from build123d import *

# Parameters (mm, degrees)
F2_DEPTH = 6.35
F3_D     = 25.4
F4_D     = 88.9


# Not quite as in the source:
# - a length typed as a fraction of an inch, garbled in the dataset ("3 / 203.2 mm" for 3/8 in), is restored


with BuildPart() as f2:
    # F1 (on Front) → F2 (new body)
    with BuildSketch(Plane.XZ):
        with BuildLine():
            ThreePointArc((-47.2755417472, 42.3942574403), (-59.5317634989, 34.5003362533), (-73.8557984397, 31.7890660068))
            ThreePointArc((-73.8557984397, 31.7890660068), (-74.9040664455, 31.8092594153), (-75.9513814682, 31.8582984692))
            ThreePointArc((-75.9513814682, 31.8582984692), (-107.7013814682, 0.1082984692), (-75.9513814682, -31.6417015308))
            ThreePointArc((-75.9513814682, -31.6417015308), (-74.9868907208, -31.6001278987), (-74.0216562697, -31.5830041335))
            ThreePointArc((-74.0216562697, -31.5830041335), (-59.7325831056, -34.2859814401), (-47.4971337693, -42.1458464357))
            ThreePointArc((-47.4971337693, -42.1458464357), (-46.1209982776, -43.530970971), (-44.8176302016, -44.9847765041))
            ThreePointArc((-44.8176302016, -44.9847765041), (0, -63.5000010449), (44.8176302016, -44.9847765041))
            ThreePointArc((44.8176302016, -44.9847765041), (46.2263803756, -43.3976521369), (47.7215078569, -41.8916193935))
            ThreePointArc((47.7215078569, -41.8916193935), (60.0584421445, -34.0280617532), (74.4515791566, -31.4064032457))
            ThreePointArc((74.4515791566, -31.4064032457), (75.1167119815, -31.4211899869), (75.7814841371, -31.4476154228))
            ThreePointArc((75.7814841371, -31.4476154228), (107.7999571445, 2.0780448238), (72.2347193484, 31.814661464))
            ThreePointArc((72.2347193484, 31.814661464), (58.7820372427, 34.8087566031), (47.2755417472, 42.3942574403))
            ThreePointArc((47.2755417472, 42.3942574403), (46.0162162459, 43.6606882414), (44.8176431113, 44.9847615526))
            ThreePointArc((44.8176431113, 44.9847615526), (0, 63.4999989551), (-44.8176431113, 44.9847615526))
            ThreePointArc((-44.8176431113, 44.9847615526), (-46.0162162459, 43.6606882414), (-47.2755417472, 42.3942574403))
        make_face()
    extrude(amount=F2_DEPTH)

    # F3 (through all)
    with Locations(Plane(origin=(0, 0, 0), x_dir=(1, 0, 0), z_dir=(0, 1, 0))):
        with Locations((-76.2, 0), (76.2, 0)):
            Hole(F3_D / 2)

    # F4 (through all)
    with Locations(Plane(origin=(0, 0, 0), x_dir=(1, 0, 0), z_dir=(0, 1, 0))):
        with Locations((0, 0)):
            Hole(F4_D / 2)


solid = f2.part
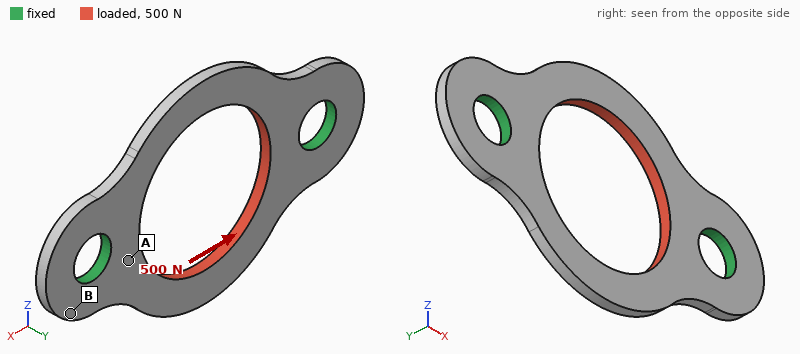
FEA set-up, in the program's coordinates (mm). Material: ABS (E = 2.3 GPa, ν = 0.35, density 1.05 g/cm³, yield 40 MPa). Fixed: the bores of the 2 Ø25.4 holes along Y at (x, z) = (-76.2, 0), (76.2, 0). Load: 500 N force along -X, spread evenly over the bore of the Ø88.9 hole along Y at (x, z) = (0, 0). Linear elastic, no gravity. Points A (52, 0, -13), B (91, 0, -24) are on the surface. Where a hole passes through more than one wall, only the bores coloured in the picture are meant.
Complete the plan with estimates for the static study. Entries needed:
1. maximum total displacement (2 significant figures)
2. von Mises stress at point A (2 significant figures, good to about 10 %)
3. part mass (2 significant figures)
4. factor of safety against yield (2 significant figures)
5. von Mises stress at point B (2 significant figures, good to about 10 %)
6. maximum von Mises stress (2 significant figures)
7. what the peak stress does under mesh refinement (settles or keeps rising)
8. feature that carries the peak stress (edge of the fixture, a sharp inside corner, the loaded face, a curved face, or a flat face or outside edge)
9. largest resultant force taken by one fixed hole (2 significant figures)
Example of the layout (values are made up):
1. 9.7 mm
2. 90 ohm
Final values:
1. 40 µm
2. 0.60 MPa
3. 71 g
4. 25
5. 0.31 MPa
6. 1.6 MPa
7. settles
8. the loaded face
9. 250 N
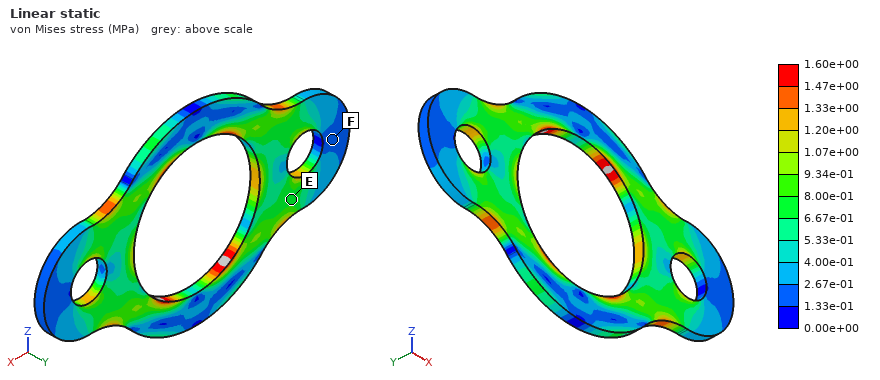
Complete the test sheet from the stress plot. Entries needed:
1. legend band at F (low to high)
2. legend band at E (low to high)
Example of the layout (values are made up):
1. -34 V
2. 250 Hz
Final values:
1. 1.33e-01 to 2.67e-01 MPa
2. 6.67e-01 to 8.00e-01 MPa
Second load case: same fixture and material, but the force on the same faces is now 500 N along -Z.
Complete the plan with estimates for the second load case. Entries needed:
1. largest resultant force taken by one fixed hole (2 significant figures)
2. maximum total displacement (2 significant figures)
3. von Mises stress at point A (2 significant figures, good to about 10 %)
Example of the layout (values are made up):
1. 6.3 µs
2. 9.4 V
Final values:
1. 250 N
2. 47 µm
3. 1.1 MPa
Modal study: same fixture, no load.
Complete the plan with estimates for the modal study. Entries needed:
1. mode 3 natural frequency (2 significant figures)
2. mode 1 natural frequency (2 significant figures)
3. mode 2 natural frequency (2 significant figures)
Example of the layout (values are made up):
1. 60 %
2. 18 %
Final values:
1. 930 Hz
2. 340 Hz
3. 350 Hz
